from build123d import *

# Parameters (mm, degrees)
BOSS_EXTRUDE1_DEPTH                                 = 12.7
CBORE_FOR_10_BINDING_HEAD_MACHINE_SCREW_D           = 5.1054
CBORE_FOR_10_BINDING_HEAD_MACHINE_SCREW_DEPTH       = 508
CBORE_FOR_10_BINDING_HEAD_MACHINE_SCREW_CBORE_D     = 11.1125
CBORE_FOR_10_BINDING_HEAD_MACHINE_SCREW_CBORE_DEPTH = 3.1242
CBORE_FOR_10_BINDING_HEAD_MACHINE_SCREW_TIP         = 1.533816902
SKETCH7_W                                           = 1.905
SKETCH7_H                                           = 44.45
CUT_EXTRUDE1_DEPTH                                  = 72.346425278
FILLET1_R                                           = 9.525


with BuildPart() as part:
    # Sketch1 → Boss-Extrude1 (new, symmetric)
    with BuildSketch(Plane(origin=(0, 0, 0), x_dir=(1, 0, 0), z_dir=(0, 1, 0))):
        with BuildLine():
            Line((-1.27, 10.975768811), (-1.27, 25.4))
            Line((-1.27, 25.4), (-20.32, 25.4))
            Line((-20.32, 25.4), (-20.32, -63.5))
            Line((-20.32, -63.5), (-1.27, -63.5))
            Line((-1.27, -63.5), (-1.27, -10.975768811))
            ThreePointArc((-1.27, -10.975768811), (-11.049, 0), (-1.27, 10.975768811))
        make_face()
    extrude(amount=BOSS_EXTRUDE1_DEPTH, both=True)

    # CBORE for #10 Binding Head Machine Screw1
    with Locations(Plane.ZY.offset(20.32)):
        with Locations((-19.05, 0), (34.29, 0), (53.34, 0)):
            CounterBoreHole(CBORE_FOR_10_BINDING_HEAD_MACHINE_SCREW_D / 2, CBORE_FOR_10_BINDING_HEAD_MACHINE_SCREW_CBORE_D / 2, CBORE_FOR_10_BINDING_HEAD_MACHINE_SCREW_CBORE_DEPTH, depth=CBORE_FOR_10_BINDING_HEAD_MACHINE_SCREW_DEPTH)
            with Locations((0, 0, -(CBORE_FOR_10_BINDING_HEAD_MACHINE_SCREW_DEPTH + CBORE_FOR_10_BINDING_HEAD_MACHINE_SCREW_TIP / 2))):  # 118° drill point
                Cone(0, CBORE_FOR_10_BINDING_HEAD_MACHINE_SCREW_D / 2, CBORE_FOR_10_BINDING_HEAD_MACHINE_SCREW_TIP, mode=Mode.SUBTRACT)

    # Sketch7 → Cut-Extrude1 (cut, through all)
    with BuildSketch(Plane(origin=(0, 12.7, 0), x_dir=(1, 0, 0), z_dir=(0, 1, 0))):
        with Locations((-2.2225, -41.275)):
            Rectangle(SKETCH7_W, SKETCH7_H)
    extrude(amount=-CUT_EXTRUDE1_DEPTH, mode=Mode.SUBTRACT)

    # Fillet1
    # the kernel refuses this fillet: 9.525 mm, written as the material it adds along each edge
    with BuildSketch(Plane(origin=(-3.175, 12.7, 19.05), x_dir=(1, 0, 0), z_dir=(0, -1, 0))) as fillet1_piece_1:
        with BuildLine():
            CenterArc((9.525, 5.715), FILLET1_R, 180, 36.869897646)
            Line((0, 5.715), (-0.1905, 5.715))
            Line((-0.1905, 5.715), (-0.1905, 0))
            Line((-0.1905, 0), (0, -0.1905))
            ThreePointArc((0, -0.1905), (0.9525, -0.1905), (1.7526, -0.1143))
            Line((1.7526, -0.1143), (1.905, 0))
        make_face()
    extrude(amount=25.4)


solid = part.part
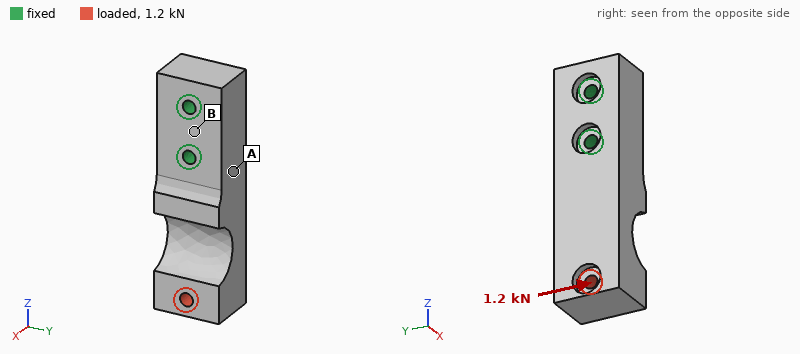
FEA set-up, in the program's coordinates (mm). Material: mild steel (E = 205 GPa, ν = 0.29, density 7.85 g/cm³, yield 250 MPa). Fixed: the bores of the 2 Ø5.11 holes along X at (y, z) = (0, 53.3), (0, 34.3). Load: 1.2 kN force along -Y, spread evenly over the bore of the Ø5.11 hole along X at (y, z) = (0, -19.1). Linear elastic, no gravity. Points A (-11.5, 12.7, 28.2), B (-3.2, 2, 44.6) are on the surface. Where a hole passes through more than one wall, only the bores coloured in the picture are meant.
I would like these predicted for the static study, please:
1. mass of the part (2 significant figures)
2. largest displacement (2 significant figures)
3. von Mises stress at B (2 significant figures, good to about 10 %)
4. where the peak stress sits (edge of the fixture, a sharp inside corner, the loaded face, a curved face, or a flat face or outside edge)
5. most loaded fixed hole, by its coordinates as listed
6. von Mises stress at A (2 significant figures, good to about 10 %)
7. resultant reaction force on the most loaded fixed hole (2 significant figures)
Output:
270 g
35 µm
11 MPa
edge of the fixture
(0, 34.3)
32 MPa
3.6 kN
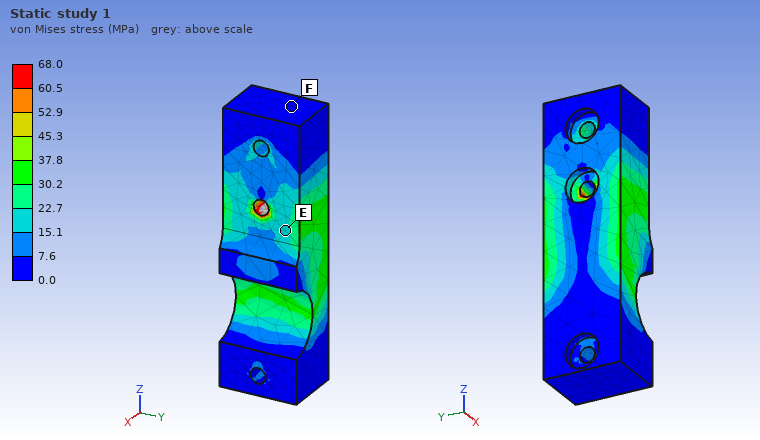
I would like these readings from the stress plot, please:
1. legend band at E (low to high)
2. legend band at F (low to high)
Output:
15.1 to 22.7 MPa
0.0 to 7.6 MPa
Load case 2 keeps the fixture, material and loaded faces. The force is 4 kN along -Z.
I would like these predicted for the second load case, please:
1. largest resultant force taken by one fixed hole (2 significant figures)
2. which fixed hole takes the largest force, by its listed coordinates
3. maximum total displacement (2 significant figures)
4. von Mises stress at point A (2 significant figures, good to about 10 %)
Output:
3.2 kN
(0, 34.3)
40 µm
6.0 MPa
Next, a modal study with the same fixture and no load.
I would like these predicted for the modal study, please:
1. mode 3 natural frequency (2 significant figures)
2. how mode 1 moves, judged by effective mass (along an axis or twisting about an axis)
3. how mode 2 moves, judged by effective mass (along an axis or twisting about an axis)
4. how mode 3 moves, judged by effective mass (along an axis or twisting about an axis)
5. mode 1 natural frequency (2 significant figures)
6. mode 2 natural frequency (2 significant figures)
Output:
9000 Hz
along X
along Y
twisting about Z
3000 Hz
4000 Hz
